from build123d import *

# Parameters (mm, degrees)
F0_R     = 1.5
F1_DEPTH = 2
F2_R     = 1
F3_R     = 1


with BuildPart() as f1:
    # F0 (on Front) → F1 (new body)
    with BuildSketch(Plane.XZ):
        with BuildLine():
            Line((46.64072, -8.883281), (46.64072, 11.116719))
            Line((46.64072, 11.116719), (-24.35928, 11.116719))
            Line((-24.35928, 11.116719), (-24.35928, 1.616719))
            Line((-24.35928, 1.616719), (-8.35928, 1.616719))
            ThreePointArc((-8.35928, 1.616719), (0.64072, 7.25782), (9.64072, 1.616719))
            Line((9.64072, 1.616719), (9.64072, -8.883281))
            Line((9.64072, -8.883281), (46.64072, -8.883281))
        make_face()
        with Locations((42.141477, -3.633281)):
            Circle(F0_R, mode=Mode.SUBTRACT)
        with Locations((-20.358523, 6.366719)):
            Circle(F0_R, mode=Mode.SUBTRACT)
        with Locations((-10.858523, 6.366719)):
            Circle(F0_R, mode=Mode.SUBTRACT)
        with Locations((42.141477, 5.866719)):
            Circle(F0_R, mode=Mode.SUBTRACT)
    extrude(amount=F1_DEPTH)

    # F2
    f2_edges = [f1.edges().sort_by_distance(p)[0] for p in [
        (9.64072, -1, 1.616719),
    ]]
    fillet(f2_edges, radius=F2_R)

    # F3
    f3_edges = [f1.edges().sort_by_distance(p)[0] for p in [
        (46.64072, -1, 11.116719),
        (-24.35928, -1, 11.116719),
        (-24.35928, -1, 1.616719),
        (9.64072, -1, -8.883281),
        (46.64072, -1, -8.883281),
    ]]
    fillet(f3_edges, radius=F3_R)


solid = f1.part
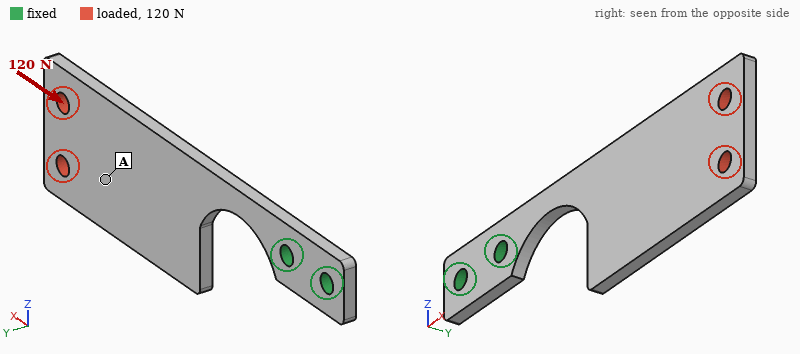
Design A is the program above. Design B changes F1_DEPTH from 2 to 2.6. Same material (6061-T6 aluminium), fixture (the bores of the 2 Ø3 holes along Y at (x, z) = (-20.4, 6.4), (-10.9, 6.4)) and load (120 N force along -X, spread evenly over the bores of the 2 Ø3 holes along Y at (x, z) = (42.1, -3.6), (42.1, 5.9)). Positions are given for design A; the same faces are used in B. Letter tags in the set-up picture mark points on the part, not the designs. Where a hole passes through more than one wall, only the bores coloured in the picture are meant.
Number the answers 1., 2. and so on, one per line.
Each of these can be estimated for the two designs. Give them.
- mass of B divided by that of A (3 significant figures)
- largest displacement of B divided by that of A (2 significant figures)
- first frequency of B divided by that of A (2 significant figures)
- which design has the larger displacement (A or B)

1. 1.30
2. 0.77
3. 1.3
4. A
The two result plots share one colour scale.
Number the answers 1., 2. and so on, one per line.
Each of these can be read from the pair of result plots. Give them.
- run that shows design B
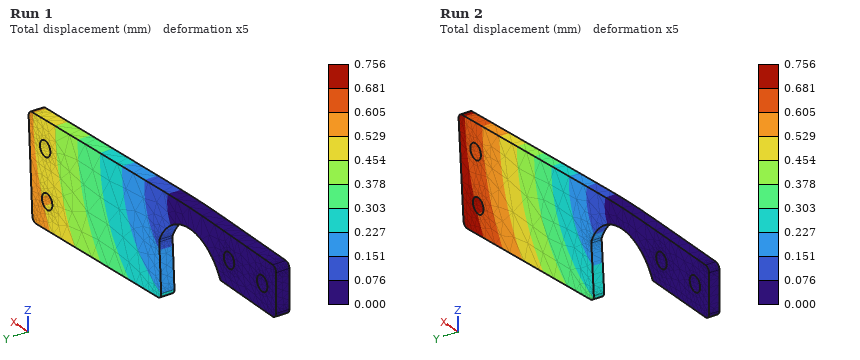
1. Run 1
